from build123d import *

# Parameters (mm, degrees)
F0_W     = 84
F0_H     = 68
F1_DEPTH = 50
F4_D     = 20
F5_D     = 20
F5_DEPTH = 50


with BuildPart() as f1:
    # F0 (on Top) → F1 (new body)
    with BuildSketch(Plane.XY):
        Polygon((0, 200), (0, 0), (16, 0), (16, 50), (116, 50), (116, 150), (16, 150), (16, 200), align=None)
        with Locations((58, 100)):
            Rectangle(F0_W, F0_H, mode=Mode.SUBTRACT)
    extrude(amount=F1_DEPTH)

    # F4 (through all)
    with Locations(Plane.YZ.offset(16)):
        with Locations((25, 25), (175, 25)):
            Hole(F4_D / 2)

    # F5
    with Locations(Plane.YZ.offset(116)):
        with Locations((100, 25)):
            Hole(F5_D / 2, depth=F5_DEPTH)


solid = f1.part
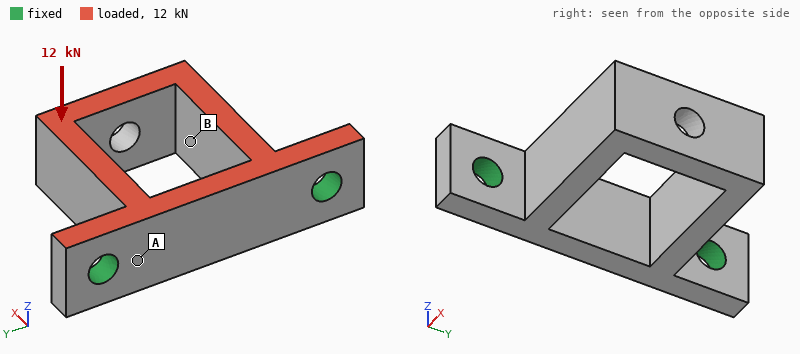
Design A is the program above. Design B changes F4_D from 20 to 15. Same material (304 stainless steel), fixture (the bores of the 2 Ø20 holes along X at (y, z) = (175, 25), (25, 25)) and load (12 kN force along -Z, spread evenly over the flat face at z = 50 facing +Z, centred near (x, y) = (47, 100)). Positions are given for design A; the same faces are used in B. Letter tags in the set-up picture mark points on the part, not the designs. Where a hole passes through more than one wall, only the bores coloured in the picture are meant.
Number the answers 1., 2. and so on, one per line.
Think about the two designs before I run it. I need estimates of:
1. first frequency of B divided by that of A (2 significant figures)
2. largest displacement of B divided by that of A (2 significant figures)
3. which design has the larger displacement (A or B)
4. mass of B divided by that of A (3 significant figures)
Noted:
1. 0.92
2. 1.2
3. B
4. 1.01
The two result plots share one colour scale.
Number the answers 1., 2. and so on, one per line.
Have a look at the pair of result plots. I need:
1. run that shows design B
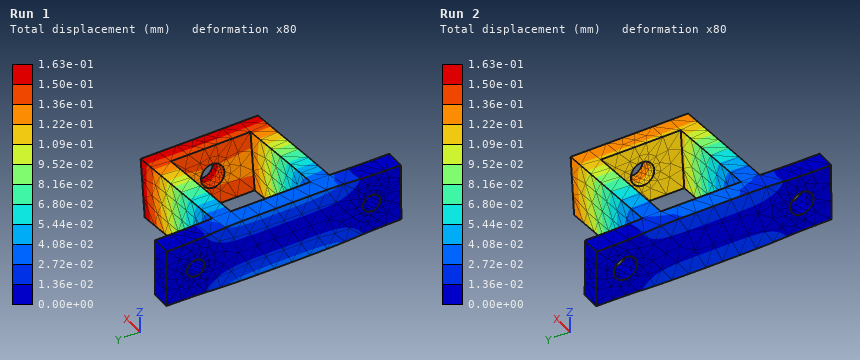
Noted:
1. Run 1
